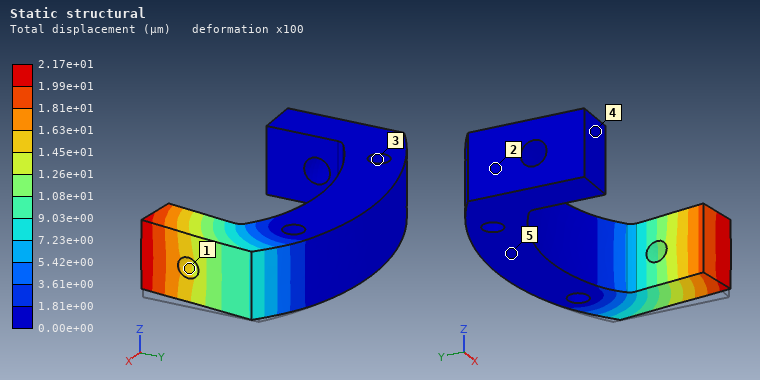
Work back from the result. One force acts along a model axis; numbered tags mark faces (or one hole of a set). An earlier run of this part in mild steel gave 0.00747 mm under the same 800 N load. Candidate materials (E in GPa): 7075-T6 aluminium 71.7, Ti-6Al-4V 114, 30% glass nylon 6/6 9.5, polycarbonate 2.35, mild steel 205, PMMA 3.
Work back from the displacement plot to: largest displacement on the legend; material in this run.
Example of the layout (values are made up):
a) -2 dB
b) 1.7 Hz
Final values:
a) 2.17e+01 µm
b) 7075-T6 aluminium
